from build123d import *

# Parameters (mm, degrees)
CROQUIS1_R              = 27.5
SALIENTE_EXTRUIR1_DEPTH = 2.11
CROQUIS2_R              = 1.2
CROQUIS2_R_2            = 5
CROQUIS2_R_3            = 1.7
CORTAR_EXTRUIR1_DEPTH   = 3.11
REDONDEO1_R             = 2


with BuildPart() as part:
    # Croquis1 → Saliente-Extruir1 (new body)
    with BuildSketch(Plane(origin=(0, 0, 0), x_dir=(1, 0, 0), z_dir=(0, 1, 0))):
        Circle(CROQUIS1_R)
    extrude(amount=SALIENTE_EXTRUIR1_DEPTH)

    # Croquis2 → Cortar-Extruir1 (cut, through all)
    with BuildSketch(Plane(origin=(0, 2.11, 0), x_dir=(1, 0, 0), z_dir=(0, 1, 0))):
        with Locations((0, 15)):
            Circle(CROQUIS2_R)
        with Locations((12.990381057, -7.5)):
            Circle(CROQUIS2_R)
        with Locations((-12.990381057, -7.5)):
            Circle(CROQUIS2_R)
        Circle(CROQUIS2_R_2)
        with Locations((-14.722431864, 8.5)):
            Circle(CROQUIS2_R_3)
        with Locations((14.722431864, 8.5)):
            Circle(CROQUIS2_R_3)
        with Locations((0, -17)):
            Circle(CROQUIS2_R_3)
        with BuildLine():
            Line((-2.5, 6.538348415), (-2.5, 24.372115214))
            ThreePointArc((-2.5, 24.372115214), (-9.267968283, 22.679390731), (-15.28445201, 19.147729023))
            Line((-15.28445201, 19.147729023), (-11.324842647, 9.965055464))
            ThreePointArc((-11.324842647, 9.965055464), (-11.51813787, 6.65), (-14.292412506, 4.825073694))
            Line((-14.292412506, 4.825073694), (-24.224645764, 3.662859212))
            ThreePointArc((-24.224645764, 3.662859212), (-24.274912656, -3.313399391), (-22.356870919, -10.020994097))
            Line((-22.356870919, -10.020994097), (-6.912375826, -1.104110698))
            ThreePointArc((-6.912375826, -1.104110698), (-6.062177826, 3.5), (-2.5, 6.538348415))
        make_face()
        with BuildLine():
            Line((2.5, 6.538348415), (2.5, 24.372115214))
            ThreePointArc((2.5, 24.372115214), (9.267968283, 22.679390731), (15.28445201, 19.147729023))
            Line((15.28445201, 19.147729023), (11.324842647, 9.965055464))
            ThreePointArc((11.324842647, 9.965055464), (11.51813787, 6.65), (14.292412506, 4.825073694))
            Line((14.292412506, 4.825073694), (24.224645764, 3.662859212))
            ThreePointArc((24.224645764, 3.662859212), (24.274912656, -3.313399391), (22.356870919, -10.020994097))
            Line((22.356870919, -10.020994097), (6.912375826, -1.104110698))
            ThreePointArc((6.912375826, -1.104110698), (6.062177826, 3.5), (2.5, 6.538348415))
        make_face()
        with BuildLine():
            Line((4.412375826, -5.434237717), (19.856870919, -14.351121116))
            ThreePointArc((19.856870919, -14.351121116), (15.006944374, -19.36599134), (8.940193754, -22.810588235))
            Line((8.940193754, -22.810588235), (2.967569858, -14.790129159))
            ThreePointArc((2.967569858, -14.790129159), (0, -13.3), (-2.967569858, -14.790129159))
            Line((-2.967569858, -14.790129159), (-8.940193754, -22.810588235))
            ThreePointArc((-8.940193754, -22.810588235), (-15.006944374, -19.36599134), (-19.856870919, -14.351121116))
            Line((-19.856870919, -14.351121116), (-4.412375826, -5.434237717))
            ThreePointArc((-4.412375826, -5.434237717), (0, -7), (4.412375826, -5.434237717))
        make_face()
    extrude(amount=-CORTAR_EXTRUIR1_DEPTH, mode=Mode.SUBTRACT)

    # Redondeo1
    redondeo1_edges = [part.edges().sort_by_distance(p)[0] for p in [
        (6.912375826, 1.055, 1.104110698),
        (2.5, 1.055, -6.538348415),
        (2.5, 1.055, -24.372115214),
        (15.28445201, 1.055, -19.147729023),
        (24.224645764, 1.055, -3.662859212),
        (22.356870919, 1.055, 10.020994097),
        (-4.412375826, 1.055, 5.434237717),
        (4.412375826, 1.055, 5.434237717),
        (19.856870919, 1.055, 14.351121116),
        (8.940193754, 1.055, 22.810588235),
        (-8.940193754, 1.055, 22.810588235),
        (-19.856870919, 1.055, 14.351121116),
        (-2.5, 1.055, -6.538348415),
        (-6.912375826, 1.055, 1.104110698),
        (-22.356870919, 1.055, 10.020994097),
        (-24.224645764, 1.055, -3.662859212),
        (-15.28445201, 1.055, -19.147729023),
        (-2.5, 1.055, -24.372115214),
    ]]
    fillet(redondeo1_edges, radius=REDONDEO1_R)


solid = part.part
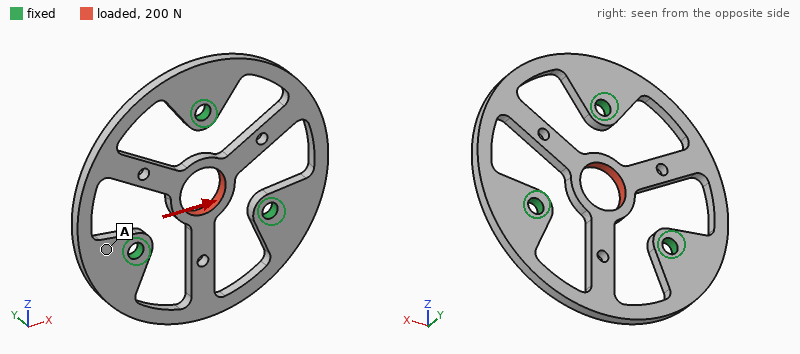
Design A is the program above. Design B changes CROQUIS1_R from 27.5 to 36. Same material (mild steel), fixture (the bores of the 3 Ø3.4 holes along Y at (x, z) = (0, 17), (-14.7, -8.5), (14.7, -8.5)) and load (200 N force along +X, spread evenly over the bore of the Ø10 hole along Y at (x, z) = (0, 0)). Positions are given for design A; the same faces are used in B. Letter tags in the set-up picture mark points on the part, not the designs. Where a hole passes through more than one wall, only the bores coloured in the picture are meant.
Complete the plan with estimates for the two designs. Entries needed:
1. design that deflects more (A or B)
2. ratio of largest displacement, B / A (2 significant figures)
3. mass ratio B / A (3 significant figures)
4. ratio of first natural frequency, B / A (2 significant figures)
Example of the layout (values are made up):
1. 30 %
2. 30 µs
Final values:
1. A
2. 0.45
3. 2.45
4. 0.74
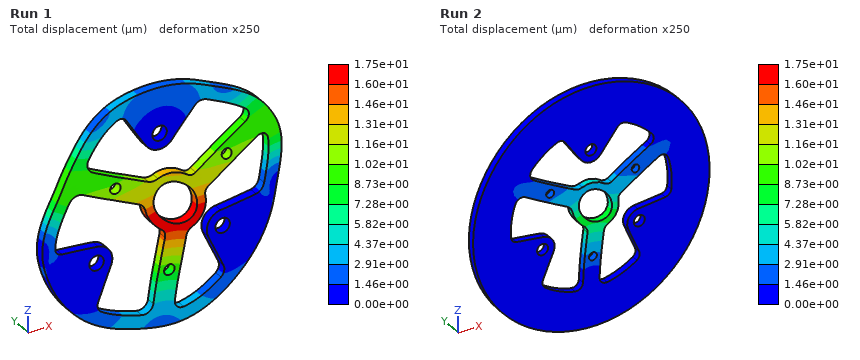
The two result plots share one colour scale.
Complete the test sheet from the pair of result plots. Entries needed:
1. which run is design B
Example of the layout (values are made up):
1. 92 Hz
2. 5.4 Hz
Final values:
1. Run 2
